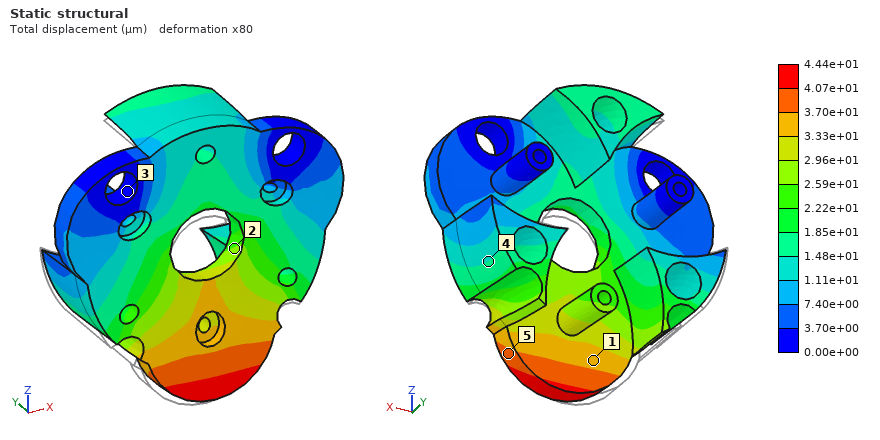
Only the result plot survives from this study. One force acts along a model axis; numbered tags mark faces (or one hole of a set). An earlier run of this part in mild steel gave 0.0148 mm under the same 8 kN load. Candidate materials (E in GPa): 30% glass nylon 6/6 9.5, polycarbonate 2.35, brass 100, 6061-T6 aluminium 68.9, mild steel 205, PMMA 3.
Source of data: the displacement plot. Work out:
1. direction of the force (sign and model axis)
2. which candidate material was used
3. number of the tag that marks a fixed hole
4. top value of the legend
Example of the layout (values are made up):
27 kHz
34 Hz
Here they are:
+Z
6061-T6 aluminium
3
4.44e+01 µm
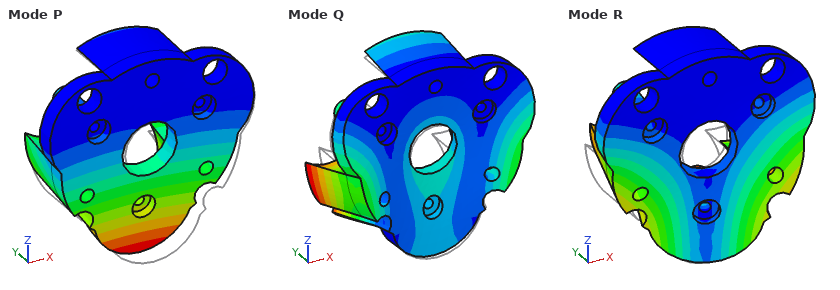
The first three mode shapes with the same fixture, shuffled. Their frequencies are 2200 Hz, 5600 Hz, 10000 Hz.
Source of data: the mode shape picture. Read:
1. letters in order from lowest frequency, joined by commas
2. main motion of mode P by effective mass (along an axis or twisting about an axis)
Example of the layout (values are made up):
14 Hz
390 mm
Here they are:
P, R, Q
along Y
